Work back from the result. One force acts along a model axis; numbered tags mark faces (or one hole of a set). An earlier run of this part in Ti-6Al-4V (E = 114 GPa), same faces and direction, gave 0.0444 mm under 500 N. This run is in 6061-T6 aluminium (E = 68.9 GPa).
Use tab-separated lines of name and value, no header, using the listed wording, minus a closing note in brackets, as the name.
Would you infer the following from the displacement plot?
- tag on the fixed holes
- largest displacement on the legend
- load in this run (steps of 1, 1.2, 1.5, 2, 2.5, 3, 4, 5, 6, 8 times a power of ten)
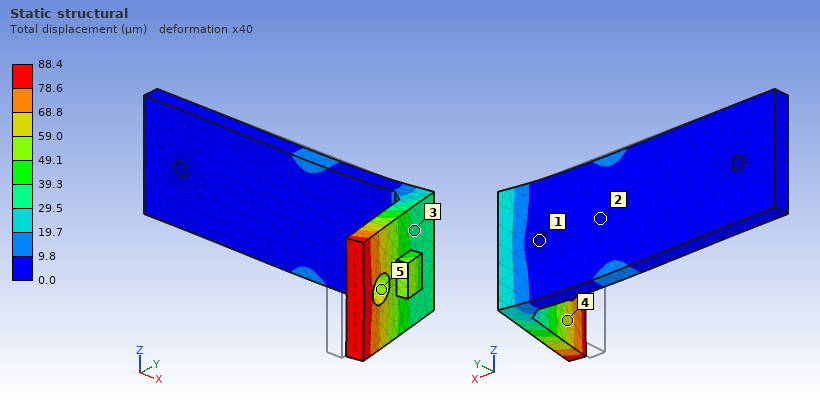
tag on the fixed holes	1
largest displacement on the legend	88.4 µm
load in this run	600 N
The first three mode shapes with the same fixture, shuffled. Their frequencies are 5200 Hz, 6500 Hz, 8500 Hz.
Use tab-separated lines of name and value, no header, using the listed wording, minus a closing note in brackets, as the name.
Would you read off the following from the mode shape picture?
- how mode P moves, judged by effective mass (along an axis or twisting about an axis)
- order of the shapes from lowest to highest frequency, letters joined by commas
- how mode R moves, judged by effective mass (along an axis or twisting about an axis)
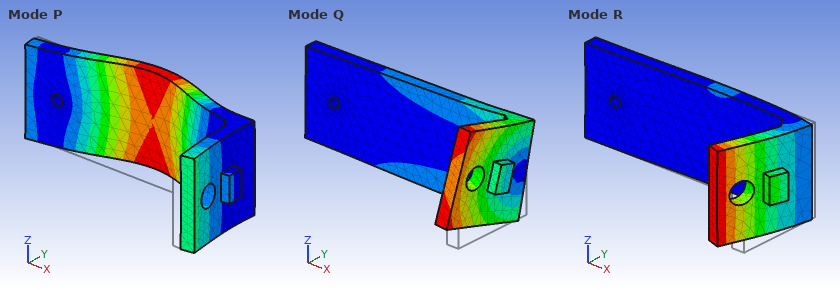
how mode P moves, judged by effective mass	along Y
order of the shapes from lowest to highest frequency, letters joined by commas	R, Q, P
how mode R moves, judged by effective mass	along X
